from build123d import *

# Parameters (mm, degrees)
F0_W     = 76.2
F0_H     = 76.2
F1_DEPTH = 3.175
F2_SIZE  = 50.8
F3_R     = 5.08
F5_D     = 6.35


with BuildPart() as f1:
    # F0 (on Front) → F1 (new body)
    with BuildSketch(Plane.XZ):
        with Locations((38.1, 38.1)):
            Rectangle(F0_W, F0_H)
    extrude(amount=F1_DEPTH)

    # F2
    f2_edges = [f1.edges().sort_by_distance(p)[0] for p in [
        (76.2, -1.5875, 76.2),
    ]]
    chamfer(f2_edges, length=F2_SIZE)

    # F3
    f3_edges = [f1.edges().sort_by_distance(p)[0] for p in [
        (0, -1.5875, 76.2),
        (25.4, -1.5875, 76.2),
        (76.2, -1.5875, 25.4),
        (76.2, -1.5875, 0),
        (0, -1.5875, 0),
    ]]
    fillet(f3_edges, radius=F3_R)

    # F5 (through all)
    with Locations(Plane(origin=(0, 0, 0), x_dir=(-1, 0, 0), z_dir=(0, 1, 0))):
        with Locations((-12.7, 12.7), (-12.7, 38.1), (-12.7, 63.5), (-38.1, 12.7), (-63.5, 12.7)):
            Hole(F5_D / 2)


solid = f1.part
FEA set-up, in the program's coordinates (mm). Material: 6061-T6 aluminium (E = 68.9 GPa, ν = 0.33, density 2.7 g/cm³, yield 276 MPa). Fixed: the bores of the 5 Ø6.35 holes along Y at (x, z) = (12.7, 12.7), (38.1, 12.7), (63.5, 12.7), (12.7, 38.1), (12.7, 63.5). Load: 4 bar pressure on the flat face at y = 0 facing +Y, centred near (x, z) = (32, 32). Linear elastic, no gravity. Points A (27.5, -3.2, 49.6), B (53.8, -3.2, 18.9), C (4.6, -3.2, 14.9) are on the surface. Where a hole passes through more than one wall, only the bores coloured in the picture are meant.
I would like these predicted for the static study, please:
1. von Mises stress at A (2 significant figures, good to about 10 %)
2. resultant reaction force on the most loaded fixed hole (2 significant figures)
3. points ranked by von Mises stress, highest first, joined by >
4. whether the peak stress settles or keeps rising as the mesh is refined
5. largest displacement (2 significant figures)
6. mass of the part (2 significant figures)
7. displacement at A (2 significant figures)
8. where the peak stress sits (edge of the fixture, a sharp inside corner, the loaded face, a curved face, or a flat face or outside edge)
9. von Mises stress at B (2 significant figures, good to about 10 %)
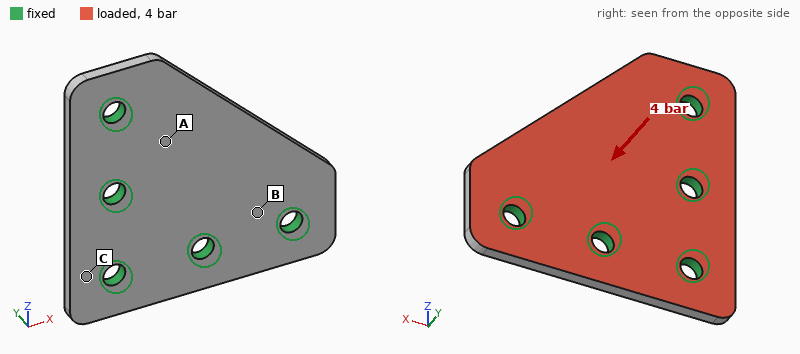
19 MPa
400 N
B > A > C
keeps rising
0.15 mm
37 g
0.042 mm
edge of the fixture
35 MPa
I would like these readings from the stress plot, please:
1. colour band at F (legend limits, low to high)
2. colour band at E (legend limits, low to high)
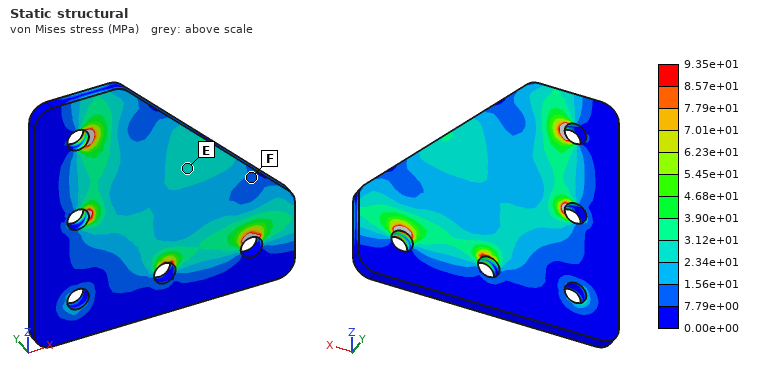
7.79e+00 to 1.56e+01 MPa
2.34e+01 to 3.12e+01 MPa
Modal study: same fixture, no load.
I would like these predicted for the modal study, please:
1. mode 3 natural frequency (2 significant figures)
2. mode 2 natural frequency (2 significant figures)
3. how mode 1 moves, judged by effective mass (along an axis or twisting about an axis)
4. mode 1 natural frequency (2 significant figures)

11 kHz
8200 Hz
along Y
3900 Hz
